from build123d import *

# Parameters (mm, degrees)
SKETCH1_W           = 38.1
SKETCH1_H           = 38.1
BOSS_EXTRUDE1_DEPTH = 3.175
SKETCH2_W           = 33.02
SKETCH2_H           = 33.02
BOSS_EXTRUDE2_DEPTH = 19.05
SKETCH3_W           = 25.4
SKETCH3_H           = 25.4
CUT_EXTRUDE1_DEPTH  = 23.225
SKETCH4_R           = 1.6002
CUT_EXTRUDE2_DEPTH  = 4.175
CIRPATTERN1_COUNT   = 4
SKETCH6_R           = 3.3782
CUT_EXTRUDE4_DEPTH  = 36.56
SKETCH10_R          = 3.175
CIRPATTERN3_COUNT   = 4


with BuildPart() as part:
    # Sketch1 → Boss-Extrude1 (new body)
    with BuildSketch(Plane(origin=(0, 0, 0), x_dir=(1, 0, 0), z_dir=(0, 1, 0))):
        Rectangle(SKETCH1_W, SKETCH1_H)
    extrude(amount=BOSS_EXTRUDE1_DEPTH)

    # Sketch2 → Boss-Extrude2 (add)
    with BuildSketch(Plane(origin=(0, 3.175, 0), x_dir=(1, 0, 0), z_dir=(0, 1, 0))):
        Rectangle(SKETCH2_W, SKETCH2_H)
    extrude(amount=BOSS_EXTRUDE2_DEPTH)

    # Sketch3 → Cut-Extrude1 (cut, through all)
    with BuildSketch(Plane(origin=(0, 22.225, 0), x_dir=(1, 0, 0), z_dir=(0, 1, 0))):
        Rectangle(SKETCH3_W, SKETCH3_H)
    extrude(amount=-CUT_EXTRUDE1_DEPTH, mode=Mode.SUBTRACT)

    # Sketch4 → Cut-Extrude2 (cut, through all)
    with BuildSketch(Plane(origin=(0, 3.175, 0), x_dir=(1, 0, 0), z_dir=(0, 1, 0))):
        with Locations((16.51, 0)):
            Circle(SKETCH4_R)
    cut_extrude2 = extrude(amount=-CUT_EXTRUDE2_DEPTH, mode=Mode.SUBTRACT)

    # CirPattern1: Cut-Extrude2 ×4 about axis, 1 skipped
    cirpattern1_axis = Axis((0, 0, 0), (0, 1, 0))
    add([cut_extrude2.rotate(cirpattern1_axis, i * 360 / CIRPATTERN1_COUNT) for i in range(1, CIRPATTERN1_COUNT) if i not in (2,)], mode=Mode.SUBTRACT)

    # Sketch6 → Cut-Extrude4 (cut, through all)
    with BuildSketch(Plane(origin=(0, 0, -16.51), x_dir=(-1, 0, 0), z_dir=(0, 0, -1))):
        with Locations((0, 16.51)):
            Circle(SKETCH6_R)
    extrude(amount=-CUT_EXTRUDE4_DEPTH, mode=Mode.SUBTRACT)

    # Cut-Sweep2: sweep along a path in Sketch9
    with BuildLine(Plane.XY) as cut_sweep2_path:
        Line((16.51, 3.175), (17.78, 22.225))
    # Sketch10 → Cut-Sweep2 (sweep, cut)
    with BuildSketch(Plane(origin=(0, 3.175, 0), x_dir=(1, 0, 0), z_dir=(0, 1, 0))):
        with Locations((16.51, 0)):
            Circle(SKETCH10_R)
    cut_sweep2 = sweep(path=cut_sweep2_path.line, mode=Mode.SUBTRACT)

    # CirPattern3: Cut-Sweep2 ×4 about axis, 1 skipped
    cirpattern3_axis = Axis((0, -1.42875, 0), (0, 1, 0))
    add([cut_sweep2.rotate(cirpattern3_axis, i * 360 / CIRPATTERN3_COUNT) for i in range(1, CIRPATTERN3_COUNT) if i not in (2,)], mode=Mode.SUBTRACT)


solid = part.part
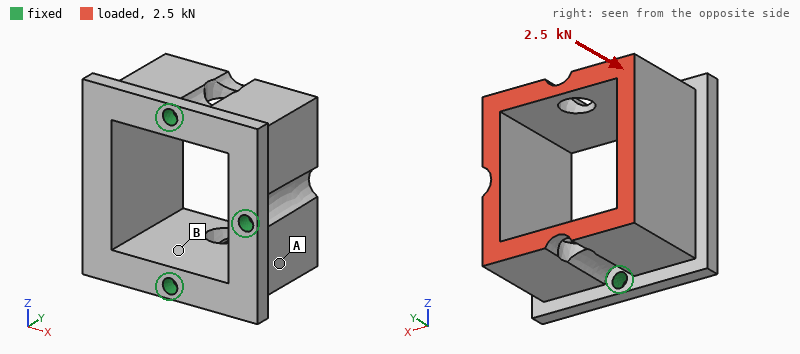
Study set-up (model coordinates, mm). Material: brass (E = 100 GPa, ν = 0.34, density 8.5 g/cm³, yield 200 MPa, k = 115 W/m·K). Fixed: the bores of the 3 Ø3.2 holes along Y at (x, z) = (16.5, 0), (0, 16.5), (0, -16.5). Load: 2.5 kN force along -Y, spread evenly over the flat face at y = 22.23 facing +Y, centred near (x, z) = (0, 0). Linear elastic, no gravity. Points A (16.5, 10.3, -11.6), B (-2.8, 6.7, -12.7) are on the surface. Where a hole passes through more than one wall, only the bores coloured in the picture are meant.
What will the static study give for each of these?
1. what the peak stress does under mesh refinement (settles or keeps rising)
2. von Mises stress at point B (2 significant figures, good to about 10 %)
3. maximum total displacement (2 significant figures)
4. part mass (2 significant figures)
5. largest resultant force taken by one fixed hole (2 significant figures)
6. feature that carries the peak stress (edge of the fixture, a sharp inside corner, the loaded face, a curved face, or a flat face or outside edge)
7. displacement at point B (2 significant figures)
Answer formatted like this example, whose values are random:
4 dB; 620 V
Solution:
keeps rising; 35 MPa; 26 µm; 86 g; 1.2 kN; edge of the fixture; 7.0 µm
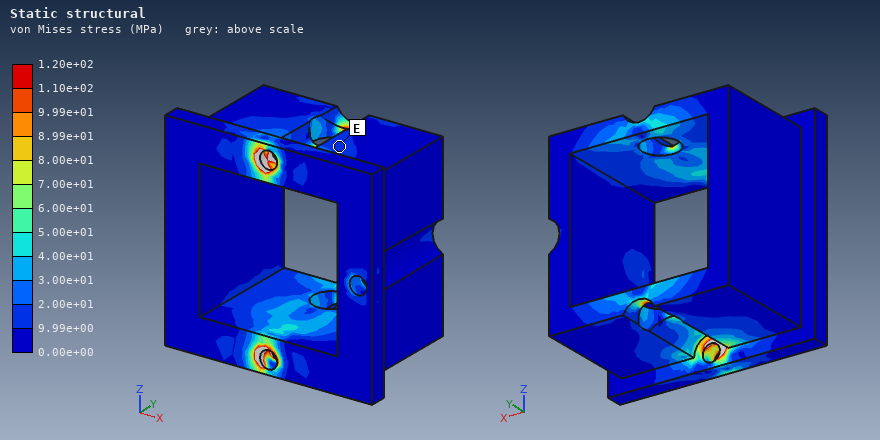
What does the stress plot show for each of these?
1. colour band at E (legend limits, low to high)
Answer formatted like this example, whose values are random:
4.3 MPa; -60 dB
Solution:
9.99e+00 to 2.00e+01 MPa
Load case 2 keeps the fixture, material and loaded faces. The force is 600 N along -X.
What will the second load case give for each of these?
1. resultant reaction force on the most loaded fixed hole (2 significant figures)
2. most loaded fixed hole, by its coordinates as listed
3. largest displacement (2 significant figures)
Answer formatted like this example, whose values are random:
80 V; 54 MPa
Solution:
680 N; (16.5, 0); 25 µm
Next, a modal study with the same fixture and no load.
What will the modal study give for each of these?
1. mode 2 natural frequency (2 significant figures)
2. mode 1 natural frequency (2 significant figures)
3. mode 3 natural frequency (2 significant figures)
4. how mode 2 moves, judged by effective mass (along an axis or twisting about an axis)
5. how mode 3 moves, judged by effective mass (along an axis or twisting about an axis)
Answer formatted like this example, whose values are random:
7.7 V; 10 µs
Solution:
5100 Hz; 4600 Hz; 5800 Hz; along Z; along Z
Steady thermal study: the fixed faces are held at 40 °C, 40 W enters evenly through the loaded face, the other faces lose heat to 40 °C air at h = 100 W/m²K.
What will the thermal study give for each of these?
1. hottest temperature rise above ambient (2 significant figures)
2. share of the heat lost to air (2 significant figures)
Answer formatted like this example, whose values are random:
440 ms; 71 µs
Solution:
31 K; 27 %
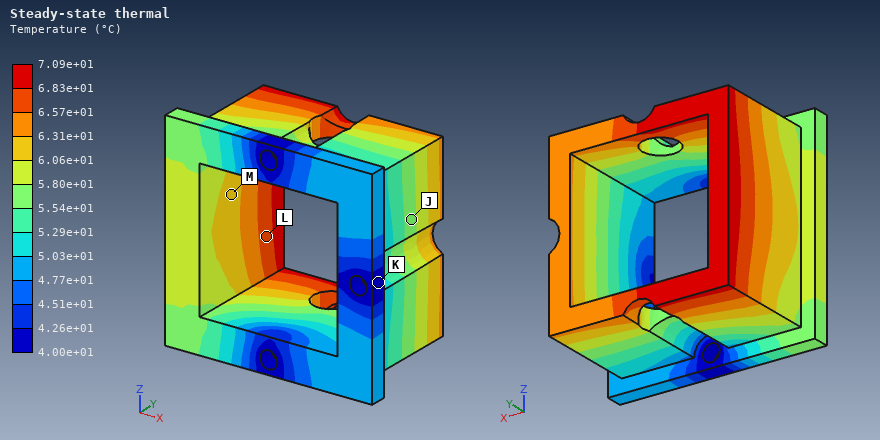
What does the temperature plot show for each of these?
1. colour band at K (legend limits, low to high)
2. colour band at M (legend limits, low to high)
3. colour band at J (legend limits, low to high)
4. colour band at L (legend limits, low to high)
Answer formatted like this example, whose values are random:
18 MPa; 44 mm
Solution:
4.00e+01 to 4.26e+01 °C; 6.06e+01 to 6.31e+01 °C; 5.54e+01 to 5.80e+01 °C; 6.57e+01 to 6.83e+01 °C
